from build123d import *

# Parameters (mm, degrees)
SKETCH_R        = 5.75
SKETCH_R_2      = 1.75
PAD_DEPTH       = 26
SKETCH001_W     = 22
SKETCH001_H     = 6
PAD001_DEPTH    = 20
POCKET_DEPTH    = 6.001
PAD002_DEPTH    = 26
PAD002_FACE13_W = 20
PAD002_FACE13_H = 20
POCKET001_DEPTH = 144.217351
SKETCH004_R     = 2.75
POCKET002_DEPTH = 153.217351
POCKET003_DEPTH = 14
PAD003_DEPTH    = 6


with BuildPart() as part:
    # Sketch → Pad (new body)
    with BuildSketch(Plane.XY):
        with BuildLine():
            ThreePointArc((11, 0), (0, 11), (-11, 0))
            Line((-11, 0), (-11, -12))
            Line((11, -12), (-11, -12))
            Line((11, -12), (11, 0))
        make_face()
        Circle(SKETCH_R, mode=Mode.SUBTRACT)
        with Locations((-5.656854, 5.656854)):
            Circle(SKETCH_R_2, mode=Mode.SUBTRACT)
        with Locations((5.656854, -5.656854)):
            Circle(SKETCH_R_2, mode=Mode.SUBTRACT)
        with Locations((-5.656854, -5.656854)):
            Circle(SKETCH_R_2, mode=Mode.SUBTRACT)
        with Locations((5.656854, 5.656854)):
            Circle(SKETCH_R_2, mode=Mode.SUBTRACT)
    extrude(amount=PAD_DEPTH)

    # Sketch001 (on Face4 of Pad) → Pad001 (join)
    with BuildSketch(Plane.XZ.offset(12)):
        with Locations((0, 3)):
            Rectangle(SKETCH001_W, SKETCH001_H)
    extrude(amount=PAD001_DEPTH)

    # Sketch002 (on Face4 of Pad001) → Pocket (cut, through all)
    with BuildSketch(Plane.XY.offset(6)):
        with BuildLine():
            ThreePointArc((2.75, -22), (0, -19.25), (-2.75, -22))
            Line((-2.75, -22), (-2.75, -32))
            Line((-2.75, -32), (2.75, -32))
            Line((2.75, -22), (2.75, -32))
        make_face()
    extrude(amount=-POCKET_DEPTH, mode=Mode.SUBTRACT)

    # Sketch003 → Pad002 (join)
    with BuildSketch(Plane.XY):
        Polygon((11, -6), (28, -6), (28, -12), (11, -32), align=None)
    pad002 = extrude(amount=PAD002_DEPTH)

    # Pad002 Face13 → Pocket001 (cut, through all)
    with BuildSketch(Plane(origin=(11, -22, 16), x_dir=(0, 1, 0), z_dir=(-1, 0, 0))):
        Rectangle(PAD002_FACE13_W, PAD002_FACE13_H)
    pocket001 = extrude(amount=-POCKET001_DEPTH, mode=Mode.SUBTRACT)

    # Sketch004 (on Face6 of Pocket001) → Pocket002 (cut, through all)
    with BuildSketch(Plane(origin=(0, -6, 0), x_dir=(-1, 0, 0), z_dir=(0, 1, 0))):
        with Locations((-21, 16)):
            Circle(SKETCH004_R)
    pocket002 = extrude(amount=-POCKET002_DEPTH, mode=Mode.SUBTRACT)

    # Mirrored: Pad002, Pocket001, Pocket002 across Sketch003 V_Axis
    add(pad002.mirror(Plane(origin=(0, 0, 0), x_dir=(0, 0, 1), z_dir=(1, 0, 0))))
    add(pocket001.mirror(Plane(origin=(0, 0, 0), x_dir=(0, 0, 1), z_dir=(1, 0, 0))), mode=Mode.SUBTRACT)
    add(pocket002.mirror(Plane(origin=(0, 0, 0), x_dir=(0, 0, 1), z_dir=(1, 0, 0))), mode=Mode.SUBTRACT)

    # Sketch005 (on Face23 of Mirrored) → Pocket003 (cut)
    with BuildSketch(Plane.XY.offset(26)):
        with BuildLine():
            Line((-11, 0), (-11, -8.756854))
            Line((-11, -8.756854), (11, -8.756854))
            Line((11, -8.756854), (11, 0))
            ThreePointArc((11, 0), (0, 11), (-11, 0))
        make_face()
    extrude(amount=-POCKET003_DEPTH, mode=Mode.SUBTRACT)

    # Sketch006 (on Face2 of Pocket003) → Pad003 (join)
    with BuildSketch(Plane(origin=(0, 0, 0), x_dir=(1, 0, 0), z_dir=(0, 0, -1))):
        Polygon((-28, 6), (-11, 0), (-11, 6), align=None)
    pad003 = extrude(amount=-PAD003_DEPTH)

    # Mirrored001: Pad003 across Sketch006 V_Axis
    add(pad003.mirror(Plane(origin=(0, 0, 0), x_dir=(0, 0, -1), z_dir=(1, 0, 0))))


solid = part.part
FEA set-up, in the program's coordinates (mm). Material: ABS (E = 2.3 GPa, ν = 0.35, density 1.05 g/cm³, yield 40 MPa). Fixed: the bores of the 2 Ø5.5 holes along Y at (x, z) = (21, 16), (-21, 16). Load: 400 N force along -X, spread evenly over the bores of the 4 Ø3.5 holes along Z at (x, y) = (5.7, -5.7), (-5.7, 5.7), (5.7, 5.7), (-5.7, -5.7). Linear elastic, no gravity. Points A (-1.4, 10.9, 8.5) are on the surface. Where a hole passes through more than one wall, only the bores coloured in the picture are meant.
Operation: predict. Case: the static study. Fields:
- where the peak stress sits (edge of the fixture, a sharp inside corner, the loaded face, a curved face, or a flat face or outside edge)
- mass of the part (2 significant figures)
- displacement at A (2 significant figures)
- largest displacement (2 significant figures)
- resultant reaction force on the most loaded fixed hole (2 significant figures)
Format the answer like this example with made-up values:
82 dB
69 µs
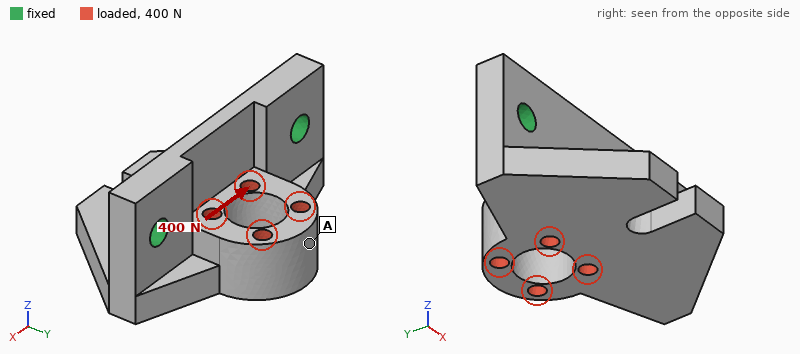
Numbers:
the loaded face
15 g
0.12 mm
0.13 mm
230 N
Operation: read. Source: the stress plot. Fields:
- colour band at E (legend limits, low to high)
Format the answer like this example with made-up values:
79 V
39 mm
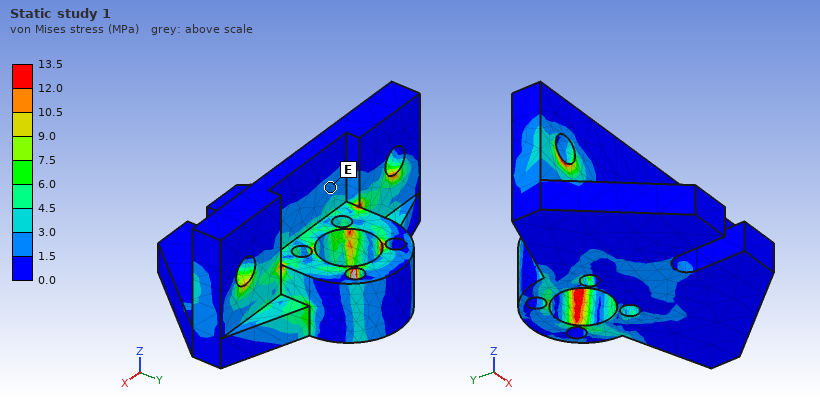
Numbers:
1.5 to 3.0 MPa
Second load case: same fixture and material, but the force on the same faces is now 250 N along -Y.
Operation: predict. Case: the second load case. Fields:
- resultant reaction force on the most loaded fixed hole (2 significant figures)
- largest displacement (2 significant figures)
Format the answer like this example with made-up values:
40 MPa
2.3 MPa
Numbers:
130 N
0.22 mm
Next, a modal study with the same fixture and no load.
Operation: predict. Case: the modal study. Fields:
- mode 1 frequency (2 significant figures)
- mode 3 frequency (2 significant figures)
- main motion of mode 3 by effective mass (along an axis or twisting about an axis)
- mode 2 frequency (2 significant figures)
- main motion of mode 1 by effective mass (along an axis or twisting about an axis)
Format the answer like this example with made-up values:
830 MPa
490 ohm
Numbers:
1500 Hz
3600 Hz
along Y
3200 Hz
along Y
